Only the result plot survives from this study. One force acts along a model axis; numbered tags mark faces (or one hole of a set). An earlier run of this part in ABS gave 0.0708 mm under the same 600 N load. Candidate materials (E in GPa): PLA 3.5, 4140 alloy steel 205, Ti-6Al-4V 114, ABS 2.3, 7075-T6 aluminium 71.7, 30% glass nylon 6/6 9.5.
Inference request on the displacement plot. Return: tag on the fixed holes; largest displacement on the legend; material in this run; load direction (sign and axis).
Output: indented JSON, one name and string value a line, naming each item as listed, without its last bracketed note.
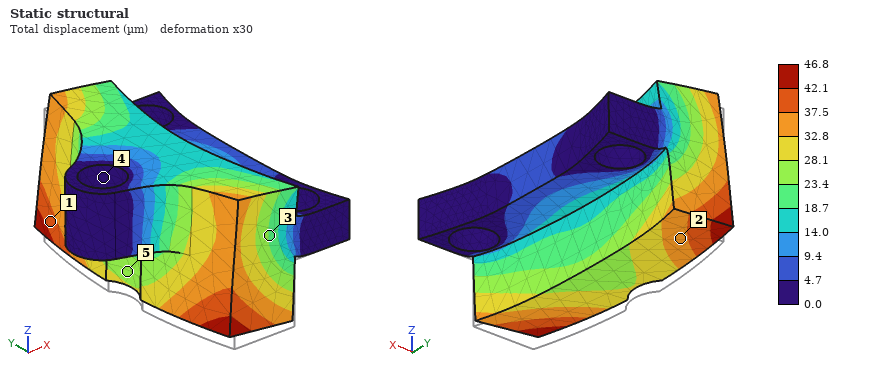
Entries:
{
  "tag on the fixed holes": "4",
  "largest displacement on the legend": "46.8 µm",
  "material in this run": "PLA",
  "load direction": "+Z"
}
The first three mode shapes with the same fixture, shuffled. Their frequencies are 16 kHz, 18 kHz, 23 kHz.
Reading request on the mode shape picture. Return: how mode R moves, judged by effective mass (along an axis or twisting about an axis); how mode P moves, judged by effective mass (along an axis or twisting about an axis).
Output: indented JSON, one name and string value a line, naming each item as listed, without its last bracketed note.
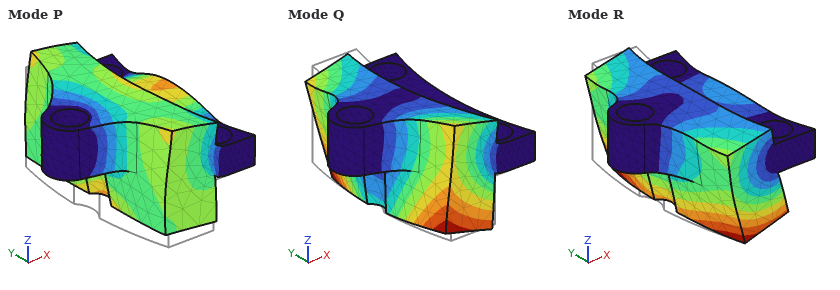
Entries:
{
  "how mode R moves, judged by effective mass": "along X",
  "how mode P moves, judged by effective mass": "along Z"
}
